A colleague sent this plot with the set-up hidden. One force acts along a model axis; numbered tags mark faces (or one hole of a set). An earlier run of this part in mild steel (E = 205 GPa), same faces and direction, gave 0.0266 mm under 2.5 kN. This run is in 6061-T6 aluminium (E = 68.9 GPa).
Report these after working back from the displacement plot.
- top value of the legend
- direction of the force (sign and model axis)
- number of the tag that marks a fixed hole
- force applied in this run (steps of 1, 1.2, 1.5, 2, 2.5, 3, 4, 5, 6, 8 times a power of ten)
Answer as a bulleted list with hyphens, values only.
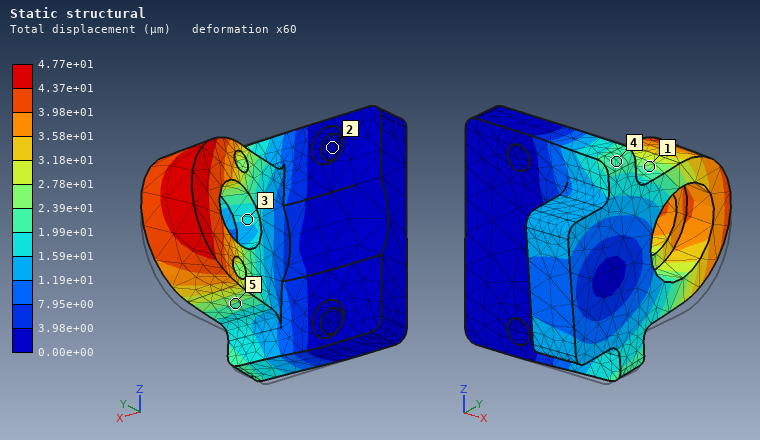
- 4.77e+01 µm
- +Z
- 2
- 1.5 kN
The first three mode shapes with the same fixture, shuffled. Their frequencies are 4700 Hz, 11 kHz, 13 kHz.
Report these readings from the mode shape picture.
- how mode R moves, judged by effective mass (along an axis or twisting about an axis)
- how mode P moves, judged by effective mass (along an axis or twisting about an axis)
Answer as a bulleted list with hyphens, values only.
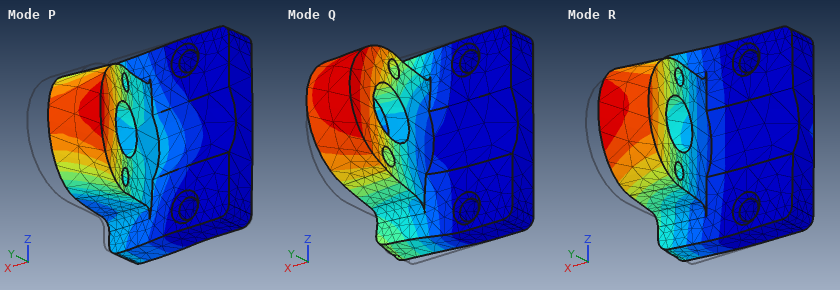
- along Y
- along Y
